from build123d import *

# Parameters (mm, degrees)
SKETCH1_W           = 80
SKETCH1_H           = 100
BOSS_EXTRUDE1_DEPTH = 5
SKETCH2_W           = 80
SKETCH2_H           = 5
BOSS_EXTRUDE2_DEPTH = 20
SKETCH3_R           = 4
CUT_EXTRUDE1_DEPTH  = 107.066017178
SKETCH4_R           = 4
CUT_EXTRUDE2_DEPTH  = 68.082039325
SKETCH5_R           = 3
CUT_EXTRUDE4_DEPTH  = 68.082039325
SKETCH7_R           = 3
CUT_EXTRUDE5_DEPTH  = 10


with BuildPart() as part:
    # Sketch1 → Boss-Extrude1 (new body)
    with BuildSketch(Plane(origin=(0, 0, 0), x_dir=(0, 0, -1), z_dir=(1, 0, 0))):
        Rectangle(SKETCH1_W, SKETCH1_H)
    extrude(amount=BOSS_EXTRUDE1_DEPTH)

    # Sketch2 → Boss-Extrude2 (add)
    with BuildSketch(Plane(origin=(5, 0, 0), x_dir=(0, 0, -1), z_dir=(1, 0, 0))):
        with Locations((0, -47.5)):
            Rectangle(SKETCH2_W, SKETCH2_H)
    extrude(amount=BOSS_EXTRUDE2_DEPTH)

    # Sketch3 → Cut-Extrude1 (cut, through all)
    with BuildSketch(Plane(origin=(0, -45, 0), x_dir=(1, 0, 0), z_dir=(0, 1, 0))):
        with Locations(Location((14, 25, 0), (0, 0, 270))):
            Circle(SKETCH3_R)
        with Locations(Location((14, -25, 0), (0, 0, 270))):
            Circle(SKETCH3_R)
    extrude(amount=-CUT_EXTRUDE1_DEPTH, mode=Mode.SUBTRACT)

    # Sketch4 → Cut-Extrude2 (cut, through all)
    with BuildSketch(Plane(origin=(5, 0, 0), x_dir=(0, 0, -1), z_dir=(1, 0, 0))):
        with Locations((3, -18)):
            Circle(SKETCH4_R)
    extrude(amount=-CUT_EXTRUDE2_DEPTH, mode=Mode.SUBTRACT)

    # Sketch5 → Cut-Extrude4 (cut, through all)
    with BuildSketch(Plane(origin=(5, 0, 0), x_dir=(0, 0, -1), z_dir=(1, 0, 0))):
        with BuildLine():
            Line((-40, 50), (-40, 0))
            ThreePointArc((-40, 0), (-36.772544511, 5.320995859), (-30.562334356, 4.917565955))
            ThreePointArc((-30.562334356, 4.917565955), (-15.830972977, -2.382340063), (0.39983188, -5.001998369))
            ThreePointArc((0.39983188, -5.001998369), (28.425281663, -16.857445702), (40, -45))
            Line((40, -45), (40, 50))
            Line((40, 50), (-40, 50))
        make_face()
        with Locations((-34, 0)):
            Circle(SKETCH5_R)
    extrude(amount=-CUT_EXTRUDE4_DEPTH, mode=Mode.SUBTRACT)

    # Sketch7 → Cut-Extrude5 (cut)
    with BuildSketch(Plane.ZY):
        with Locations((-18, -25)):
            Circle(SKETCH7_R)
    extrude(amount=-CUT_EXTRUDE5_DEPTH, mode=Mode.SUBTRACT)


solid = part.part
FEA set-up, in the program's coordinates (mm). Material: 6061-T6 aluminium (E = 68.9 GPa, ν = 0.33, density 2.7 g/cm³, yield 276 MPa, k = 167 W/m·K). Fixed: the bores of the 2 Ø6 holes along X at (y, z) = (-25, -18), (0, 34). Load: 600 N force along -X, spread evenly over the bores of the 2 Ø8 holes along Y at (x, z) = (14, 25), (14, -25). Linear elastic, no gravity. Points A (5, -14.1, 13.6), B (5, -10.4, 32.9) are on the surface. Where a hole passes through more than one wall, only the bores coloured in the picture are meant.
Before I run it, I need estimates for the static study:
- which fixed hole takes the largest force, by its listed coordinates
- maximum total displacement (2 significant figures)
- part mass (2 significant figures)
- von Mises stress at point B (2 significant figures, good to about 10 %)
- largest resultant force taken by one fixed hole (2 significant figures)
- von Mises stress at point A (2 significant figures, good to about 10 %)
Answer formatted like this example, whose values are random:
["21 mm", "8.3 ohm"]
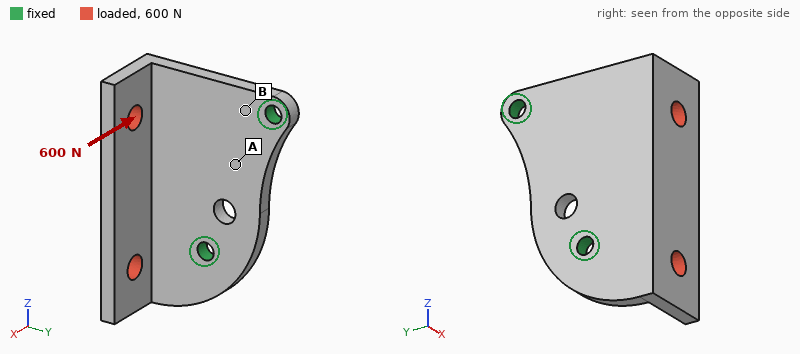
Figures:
["(-25, -18)", "0.25 mm", "65 g", "37 MPa", "510 N", "15 MPa"]
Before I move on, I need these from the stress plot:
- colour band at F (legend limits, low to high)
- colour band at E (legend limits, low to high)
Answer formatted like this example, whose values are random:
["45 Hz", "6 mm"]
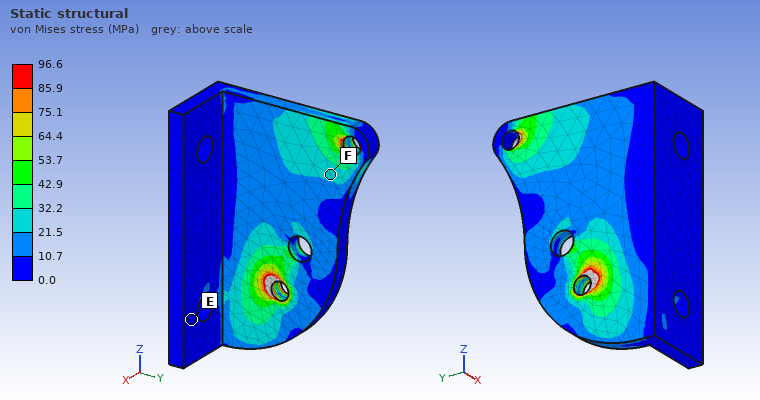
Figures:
["21.5 to 32.2 MPa", "0.0 to 10.7 MPa"]
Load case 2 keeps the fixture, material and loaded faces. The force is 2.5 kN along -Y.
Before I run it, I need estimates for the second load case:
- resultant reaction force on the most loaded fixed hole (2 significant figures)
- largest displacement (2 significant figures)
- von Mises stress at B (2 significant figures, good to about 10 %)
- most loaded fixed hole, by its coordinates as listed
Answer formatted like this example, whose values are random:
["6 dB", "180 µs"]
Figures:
["1.6 kN", "0.55 mm", "59 MPa", "(-25, -18)"]
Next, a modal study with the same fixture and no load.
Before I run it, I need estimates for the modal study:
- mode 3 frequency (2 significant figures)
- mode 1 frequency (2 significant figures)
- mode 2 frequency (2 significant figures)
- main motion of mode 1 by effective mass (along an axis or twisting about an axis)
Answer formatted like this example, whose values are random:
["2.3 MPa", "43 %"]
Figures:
["5300 Hz", "1600 Hz", "2900 Hz", "along X"]
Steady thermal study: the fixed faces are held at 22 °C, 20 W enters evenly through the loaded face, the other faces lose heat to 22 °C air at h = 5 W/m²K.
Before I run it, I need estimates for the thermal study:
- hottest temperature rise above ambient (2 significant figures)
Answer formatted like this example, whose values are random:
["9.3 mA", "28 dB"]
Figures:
["18 K"]
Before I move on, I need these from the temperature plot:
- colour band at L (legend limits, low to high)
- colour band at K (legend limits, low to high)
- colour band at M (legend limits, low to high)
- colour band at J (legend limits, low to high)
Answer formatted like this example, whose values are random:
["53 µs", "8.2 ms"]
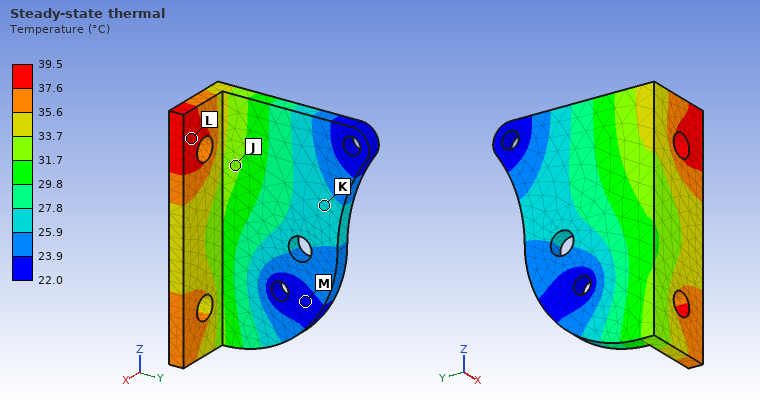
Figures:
["37.6 to 39.5 °C", "25.9 to 27.8 °C", "22.0 to 23.9 °C", "31.7 to 33.7 °C"]
